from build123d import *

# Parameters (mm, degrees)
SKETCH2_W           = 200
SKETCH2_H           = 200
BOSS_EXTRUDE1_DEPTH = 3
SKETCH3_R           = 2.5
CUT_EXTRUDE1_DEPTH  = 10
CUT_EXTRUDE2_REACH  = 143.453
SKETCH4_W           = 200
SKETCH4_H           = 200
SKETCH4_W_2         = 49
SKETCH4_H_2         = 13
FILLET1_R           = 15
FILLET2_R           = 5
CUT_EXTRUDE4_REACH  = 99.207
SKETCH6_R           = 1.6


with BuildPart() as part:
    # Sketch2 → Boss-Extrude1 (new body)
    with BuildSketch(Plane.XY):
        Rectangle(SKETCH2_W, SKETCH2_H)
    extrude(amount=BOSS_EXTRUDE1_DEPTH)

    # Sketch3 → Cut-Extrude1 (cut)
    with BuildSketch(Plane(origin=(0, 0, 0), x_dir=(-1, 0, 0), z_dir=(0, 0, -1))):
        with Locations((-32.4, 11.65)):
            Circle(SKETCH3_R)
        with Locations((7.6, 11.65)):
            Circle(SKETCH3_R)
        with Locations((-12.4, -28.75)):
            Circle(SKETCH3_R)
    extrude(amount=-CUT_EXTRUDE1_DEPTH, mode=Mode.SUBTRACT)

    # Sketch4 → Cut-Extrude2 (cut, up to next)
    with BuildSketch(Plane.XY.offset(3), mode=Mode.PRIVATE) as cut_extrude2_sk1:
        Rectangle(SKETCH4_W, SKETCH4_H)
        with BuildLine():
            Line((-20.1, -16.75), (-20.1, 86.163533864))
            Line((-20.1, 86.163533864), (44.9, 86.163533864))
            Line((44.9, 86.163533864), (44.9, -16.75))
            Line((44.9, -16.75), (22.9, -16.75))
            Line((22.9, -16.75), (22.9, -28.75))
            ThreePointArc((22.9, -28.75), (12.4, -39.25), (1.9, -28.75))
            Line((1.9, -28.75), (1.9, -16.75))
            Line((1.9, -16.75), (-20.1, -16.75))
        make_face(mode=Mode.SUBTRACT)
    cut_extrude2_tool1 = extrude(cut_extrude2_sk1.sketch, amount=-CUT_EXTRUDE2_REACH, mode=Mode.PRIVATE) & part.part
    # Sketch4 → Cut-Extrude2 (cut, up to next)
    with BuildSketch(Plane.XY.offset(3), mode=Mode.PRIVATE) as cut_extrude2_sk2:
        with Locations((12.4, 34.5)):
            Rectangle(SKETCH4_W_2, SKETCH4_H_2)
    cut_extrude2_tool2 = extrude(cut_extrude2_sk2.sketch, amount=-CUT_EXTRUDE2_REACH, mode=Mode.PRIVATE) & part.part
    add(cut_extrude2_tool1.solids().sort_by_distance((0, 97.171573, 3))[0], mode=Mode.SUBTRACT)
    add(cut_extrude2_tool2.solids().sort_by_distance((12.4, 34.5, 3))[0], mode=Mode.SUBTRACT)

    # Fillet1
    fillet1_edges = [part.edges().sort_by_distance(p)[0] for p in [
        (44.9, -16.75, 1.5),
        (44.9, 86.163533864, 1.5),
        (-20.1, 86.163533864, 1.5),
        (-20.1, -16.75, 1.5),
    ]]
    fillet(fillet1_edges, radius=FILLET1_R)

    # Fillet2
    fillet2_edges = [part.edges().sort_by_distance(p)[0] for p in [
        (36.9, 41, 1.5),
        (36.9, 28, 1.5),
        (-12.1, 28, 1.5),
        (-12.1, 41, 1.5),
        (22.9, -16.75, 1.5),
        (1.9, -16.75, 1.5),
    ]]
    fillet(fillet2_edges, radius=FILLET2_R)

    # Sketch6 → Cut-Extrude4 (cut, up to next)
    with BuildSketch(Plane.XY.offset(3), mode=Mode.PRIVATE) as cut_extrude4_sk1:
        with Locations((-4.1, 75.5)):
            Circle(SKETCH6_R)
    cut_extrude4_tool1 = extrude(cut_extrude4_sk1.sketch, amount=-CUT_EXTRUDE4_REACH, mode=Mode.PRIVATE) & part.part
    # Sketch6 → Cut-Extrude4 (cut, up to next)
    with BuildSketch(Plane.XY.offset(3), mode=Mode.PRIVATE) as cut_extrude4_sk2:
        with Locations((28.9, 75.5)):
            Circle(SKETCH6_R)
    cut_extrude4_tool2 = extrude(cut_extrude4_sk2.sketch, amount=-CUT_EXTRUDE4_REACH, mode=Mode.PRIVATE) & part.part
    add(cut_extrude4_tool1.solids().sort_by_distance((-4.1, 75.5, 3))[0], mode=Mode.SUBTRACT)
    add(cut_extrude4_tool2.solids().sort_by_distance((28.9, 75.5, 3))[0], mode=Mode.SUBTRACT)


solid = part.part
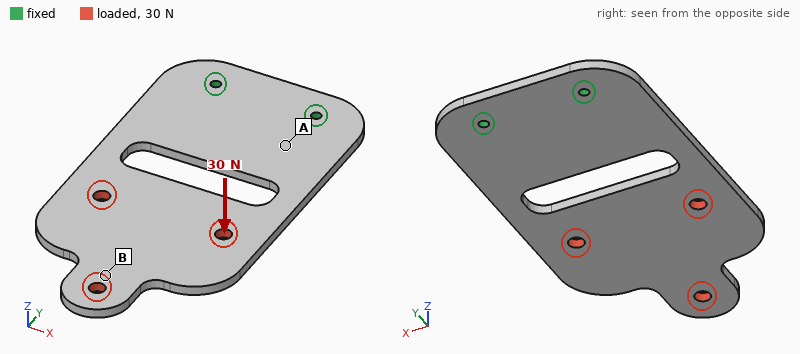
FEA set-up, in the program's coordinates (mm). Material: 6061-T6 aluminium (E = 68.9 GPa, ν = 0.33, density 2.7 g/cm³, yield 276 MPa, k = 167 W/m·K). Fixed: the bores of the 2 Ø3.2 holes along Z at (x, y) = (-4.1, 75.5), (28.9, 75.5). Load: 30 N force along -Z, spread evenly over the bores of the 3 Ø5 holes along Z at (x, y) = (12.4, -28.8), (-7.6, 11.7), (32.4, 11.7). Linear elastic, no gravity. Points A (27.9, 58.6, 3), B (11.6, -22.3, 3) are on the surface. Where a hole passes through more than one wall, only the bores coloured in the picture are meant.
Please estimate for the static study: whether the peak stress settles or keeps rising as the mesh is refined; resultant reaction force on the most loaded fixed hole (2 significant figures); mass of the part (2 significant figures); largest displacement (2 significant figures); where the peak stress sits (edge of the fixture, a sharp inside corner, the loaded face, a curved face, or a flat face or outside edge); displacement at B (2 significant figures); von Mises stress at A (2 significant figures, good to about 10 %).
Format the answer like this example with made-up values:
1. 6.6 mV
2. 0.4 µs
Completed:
1. keeps rising
2. 15 N
3. 51 g
4. 1.4 mm
5. edge of the fixture
6. 1.1 mm
7. 16 MPa
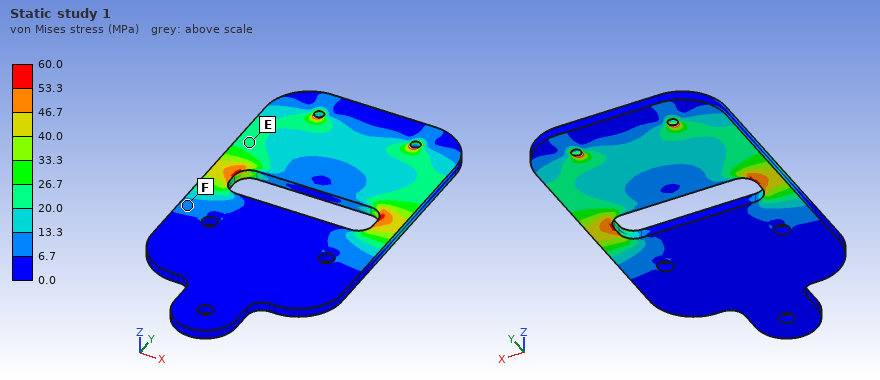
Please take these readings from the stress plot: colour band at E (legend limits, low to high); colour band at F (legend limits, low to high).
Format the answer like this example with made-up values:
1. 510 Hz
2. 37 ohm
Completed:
1. 20.0 to 26.7 MPa
2. 6.7 to 13.3 MPa
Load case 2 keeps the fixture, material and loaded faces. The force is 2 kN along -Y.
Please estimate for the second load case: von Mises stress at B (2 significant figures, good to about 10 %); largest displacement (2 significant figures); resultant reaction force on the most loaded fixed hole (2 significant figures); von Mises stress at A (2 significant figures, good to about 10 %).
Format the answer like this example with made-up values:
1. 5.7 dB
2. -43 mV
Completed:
1. 11 MPa
2. 39 µm
3. 1.0 kN
4. 13 MPa
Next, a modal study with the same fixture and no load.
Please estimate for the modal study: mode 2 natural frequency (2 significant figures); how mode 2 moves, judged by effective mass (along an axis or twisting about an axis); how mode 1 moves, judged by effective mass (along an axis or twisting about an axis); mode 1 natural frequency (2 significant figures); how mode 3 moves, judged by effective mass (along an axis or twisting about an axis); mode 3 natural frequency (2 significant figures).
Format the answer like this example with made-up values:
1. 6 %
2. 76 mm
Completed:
1. 850 Hz
2. twisting about Y
3. along Z
4. 200 Hz
5. along Z
6. 1200 Hz
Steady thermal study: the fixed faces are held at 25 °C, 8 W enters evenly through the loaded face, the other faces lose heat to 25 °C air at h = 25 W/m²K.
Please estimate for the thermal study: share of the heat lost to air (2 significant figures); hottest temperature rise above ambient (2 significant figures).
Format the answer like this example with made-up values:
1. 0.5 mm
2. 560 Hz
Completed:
1. 50 %
2. 25 K
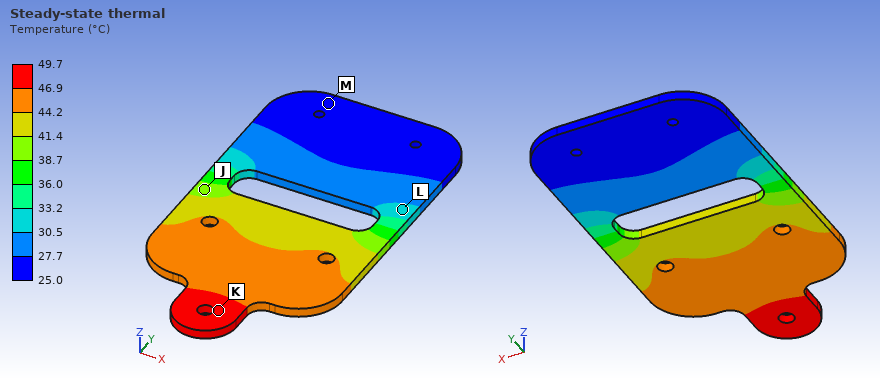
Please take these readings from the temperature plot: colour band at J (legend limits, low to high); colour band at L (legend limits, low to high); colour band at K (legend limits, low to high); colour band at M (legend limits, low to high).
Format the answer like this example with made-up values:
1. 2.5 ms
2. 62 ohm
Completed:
1. 38.7 to 41.4 °C
2. 30.5 to 33.2 °C
3. 46.9 to 49.7 °C
4. 25.0 to 27.7 °C
